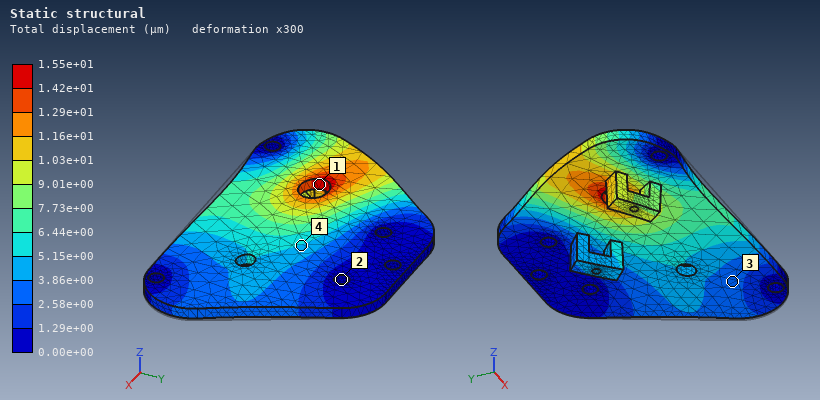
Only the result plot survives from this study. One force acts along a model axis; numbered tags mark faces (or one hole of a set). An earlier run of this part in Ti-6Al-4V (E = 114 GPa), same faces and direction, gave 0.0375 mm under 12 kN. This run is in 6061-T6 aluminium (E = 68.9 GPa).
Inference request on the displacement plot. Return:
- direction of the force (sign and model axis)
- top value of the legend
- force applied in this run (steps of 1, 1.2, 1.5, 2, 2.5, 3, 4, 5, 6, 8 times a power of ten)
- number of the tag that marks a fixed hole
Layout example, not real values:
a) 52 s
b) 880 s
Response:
a) -X
b) 1.55e+01 µm
c) 3 kN
d) 2
